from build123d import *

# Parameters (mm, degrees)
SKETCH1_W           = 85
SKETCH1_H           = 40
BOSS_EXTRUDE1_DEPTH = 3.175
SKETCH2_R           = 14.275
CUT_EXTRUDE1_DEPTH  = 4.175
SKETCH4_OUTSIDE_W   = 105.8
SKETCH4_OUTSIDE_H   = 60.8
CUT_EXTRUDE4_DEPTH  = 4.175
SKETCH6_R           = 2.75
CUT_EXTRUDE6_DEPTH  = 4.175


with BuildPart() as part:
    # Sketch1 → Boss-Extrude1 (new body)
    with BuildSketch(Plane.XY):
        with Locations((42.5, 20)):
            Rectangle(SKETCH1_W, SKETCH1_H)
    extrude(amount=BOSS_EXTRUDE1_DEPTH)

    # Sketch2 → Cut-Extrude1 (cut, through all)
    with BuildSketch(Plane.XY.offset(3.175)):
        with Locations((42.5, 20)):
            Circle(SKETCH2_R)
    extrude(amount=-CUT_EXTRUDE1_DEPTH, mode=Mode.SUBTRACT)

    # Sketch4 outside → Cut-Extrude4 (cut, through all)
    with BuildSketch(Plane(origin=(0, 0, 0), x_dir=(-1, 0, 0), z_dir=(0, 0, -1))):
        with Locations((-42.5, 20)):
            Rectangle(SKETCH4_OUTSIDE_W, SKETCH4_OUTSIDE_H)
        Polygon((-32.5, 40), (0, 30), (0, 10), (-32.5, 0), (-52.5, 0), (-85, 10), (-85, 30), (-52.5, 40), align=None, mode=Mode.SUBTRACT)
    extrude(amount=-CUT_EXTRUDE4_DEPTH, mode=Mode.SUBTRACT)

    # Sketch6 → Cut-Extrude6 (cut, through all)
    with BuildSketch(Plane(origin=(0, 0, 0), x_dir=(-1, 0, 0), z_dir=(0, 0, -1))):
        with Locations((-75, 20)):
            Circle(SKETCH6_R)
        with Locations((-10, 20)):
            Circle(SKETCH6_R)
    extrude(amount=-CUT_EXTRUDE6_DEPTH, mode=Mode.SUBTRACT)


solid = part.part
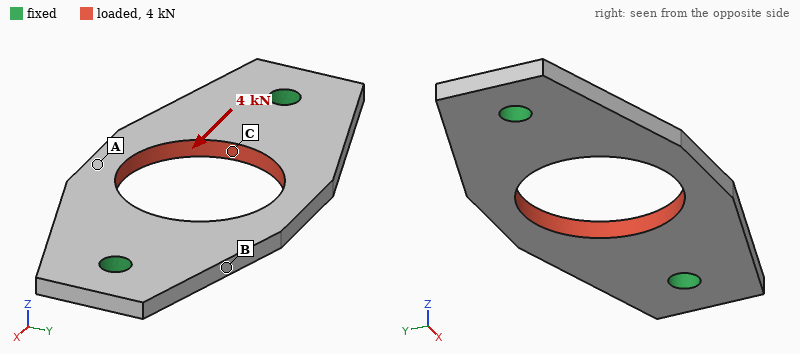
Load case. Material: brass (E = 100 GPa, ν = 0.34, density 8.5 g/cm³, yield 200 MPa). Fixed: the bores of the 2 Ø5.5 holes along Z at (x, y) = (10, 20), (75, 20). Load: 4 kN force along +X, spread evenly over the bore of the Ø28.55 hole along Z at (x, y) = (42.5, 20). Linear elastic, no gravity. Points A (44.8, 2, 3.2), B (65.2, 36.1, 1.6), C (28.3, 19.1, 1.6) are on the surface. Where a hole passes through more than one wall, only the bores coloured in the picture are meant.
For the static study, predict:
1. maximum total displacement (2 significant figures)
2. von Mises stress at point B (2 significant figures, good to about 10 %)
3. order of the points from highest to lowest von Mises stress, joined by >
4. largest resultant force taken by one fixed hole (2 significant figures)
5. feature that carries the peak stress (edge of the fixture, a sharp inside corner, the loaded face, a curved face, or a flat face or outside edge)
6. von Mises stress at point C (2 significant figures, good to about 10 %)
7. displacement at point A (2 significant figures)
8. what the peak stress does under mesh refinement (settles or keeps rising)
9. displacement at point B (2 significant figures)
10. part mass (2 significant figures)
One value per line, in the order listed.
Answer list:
11 µm
20 MPa
C > B > A
2.0 kN
edge of the fixture
38 MPa
8.2 µm
keeps rising
6.4 µm
56 g
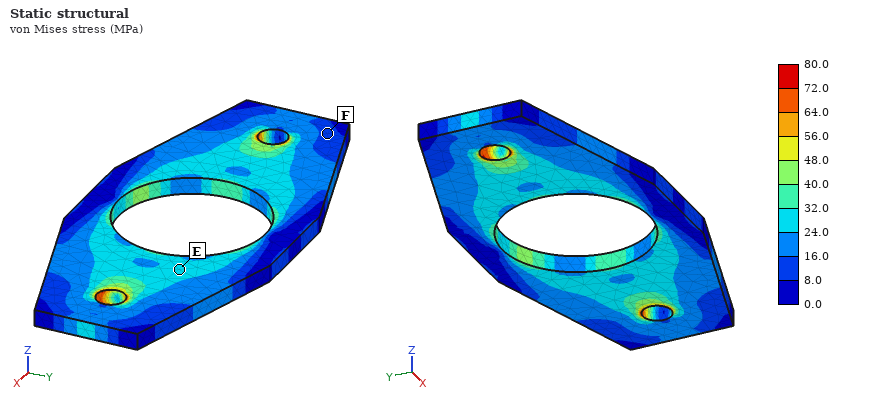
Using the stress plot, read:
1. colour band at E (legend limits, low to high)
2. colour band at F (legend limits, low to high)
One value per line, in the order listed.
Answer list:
24.0 to 32.0 MPa
8.0 to 16.0 MPa
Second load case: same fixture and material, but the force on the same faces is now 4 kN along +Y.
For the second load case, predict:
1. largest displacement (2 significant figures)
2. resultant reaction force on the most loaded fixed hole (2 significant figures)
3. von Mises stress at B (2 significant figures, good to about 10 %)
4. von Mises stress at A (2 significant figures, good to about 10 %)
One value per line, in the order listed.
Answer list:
29 µm
2.0 kN
29 MPa
68 MPa
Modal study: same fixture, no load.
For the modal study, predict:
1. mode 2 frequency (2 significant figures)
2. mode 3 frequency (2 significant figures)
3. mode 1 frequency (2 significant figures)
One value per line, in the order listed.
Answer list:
2700 Hz
5700 Hz
2600 Hz
